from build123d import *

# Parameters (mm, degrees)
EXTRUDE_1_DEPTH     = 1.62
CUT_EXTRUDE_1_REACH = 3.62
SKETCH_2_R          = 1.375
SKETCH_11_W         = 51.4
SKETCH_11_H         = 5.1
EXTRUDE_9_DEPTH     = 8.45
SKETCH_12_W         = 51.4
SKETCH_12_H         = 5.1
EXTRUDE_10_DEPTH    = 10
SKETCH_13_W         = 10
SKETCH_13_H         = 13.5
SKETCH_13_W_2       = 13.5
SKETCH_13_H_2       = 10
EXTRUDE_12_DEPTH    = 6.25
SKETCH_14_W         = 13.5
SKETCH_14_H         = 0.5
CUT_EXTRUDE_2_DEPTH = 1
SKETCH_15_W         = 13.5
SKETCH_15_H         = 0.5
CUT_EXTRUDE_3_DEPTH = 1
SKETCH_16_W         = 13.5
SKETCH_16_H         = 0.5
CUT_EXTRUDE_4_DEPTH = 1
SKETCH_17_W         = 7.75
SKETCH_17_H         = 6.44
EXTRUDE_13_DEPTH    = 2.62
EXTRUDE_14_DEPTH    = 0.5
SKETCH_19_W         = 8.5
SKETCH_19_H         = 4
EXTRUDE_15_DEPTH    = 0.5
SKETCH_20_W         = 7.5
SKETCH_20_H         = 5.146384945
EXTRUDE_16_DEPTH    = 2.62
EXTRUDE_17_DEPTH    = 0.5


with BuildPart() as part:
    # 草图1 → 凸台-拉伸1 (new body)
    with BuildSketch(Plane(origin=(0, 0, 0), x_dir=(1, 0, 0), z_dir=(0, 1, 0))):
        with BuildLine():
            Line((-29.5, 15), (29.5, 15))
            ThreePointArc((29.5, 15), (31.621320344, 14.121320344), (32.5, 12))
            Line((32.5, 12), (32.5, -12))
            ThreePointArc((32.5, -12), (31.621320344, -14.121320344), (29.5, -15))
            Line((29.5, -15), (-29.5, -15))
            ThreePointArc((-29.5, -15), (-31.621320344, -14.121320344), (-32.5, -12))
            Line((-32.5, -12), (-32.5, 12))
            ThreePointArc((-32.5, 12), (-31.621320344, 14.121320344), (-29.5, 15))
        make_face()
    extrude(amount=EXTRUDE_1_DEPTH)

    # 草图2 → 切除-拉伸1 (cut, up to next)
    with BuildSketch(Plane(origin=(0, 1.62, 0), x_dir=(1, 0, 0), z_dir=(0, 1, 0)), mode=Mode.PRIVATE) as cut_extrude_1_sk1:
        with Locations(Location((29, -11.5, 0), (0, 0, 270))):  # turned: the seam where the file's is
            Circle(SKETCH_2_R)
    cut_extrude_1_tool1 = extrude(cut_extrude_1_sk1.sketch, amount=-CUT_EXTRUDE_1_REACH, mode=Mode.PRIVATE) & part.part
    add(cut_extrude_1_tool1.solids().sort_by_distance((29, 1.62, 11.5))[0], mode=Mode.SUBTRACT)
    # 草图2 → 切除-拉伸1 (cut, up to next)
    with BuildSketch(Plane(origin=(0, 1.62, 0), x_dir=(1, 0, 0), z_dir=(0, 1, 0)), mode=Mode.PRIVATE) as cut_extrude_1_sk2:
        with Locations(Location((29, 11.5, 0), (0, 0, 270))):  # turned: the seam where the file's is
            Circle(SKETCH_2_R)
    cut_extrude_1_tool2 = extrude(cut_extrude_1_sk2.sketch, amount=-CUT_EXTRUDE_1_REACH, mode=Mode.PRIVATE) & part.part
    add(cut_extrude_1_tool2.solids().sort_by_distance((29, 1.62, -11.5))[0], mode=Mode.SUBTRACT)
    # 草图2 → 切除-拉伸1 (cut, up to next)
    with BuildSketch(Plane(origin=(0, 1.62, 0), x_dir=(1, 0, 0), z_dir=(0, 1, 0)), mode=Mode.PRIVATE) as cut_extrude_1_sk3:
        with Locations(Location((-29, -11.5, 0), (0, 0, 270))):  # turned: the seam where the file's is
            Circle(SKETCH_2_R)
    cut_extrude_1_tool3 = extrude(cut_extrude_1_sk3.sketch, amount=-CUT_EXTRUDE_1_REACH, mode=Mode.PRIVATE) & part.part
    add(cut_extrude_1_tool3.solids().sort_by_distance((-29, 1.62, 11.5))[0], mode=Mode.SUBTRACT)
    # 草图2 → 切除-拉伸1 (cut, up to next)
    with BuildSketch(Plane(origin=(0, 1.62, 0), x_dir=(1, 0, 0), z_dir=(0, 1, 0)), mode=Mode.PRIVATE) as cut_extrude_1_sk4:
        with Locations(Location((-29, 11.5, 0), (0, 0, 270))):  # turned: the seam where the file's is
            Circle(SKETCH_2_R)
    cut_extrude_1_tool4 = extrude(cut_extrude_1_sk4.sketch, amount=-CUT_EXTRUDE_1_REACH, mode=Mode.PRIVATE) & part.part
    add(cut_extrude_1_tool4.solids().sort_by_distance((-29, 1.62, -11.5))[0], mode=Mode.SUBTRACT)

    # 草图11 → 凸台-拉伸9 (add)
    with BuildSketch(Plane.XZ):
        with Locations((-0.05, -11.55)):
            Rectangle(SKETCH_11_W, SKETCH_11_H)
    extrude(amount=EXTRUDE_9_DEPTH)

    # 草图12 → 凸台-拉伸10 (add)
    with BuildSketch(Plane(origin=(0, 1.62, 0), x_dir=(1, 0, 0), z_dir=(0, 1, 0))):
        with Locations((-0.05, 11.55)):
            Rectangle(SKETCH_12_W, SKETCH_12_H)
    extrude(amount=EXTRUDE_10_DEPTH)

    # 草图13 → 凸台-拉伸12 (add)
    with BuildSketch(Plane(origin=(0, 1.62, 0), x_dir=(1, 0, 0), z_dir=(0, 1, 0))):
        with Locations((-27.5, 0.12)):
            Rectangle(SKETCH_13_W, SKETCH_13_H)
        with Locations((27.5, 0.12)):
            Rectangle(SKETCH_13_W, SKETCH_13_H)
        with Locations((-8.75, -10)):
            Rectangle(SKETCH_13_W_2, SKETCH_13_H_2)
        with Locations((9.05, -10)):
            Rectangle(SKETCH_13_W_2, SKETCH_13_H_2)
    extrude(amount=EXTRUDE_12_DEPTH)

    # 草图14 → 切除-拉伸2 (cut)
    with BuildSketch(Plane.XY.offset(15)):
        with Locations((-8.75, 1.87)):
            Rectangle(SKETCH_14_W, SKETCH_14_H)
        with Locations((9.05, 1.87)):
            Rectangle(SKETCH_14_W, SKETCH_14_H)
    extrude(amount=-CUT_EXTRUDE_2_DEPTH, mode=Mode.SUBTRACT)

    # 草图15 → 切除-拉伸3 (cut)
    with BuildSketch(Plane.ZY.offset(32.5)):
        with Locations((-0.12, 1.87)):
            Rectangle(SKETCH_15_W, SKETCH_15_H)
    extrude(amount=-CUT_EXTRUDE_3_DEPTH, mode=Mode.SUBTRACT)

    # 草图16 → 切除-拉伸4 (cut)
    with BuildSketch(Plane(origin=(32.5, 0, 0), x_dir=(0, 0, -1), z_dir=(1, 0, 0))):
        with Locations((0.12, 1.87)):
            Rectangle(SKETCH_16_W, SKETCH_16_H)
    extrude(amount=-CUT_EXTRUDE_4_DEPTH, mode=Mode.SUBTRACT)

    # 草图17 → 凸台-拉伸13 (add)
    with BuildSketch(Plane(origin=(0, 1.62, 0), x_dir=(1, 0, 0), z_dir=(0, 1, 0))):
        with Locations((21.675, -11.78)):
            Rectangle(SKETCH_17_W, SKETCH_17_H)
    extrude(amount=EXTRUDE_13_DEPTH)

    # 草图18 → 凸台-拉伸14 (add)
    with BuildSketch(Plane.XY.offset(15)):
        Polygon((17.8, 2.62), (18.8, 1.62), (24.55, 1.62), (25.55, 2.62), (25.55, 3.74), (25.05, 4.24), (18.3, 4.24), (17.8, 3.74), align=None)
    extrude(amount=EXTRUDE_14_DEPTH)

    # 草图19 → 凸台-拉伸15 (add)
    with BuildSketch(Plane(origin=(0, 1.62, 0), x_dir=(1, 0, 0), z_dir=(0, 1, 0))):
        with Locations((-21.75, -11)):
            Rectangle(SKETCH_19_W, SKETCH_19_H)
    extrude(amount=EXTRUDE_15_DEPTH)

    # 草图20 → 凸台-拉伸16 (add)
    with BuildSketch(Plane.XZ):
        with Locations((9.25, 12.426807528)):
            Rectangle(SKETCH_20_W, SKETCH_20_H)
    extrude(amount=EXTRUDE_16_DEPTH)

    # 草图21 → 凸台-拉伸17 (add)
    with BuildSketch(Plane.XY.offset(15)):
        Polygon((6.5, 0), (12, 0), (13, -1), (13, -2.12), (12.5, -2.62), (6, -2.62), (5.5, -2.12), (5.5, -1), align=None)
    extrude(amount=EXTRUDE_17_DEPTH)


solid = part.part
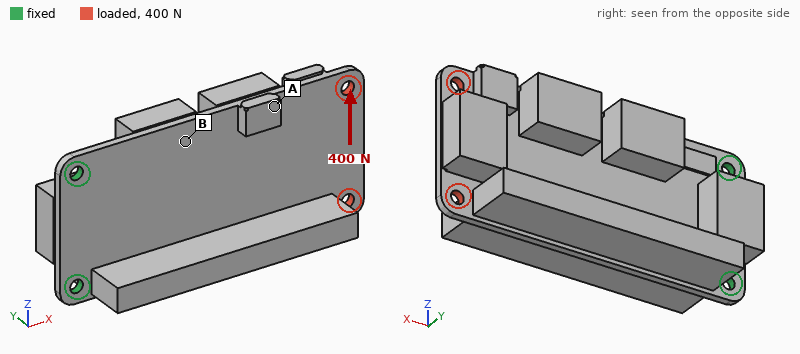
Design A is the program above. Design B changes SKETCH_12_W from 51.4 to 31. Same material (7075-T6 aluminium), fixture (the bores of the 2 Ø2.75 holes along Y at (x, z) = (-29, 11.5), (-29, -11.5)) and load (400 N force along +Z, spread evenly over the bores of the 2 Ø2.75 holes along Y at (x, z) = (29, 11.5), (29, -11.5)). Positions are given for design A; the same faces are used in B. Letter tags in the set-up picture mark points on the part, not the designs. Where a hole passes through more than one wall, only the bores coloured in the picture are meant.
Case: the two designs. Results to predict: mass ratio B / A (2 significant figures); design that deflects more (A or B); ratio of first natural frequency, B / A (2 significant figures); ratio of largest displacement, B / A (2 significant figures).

0.91
B
1.0
1.6
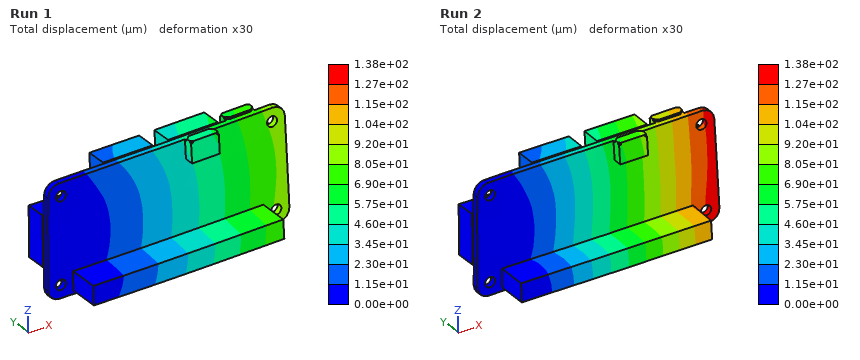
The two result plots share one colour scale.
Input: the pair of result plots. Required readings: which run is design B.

Run 2
